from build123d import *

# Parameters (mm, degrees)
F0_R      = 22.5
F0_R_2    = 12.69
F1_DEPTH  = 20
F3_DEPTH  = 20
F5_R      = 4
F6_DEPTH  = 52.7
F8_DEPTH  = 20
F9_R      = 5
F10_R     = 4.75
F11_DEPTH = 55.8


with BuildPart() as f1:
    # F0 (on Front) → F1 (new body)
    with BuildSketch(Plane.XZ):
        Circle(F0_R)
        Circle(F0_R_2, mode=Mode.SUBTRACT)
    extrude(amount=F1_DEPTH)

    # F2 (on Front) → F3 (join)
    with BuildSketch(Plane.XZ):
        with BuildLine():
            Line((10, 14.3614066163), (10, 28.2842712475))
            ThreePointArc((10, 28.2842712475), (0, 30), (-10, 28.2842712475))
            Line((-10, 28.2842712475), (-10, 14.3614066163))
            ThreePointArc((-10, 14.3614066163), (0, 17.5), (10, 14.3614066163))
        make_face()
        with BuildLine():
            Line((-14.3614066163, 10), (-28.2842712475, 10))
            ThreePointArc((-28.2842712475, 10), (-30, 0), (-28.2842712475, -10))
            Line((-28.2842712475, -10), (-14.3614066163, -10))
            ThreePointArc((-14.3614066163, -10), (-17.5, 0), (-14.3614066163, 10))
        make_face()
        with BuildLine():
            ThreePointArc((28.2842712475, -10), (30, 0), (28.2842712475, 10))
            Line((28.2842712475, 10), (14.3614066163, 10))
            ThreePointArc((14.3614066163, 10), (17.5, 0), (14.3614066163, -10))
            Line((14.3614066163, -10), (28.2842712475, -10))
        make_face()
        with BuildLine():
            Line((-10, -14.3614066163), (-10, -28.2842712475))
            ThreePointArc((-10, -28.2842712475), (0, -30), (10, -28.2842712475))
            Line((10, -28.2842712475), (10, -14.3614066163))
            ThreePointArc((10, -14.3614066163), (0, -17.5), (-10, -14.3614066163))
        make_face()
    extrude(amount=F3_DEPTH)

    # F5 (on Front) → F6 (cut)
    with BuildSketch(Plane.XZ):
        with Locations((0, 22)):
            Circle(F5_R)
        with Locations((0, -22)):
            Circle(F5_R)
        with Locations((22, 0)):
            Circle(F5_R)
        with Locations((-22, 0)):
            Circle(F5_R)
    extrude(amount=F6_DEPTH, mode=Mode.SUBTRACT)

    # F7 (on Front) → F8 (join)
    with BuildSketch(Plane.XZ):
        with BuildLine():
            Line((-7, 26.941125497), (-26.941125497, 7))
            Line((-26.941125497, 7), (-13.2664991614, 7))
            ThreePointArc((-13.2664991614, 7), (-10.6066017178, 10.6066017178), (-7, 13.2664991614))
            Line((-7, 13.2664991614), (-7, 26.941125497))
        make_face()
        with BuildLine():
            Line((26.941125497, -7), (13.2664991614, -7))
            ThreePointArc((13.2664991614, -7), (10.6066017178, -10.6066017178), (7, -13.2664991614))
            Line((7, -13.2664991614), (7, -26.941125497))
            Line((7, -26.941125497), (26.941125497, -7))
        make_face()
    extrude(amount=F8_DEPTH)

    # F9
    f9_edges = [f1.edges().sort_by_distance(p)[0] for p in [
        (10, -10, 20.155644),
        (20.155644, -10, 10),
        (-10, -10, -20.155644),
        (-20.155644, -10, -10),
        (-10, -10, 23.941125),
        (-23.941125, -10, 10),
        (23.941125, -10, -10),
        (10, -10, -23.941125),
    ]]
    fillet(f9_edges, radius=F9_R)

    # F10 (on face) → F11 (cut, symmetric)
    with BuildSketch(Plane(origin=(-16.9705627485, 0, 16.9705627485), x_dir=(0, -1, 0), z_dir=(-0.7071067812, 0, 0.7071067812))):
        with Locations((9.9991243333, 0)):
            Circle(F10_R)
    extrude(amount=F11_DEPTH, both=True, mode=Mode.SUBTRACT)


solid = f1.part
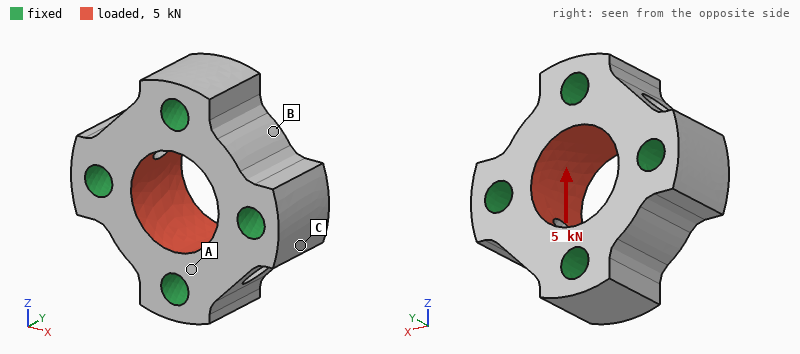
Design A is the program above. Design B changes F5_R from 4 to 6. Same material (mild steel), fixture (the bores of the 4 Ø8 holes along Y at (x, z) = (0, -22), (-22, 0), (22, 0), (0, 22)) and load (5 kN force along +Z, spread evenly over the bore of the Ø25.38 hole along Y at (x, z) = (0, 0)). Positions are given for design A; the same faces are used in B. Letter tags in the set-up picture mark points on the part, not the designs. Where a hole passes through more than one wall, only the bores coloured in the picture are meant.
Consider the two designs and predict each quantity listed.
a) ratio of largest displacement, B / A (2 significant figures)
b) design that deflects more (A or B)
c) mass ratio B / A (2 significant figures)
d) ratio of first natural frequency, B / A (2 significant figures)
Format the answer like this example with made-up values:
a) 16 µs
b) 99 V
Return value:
a) 0.70
b) A
c) 0.83
d) 1.4
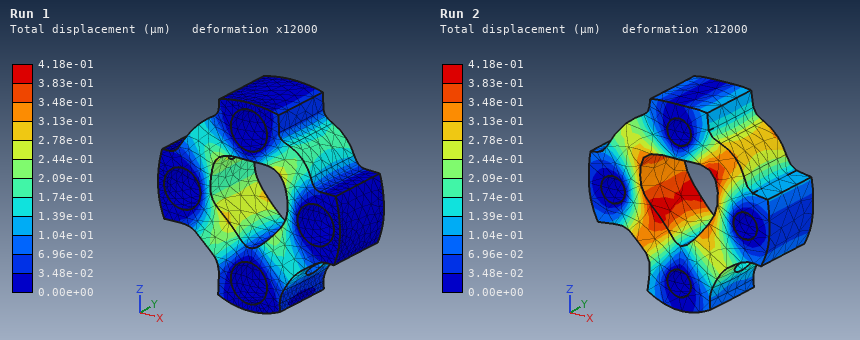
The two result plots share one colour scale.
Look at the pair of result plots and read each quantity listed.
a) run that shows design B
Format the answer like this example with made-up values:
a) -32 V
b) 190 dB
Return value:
a) Run 1
